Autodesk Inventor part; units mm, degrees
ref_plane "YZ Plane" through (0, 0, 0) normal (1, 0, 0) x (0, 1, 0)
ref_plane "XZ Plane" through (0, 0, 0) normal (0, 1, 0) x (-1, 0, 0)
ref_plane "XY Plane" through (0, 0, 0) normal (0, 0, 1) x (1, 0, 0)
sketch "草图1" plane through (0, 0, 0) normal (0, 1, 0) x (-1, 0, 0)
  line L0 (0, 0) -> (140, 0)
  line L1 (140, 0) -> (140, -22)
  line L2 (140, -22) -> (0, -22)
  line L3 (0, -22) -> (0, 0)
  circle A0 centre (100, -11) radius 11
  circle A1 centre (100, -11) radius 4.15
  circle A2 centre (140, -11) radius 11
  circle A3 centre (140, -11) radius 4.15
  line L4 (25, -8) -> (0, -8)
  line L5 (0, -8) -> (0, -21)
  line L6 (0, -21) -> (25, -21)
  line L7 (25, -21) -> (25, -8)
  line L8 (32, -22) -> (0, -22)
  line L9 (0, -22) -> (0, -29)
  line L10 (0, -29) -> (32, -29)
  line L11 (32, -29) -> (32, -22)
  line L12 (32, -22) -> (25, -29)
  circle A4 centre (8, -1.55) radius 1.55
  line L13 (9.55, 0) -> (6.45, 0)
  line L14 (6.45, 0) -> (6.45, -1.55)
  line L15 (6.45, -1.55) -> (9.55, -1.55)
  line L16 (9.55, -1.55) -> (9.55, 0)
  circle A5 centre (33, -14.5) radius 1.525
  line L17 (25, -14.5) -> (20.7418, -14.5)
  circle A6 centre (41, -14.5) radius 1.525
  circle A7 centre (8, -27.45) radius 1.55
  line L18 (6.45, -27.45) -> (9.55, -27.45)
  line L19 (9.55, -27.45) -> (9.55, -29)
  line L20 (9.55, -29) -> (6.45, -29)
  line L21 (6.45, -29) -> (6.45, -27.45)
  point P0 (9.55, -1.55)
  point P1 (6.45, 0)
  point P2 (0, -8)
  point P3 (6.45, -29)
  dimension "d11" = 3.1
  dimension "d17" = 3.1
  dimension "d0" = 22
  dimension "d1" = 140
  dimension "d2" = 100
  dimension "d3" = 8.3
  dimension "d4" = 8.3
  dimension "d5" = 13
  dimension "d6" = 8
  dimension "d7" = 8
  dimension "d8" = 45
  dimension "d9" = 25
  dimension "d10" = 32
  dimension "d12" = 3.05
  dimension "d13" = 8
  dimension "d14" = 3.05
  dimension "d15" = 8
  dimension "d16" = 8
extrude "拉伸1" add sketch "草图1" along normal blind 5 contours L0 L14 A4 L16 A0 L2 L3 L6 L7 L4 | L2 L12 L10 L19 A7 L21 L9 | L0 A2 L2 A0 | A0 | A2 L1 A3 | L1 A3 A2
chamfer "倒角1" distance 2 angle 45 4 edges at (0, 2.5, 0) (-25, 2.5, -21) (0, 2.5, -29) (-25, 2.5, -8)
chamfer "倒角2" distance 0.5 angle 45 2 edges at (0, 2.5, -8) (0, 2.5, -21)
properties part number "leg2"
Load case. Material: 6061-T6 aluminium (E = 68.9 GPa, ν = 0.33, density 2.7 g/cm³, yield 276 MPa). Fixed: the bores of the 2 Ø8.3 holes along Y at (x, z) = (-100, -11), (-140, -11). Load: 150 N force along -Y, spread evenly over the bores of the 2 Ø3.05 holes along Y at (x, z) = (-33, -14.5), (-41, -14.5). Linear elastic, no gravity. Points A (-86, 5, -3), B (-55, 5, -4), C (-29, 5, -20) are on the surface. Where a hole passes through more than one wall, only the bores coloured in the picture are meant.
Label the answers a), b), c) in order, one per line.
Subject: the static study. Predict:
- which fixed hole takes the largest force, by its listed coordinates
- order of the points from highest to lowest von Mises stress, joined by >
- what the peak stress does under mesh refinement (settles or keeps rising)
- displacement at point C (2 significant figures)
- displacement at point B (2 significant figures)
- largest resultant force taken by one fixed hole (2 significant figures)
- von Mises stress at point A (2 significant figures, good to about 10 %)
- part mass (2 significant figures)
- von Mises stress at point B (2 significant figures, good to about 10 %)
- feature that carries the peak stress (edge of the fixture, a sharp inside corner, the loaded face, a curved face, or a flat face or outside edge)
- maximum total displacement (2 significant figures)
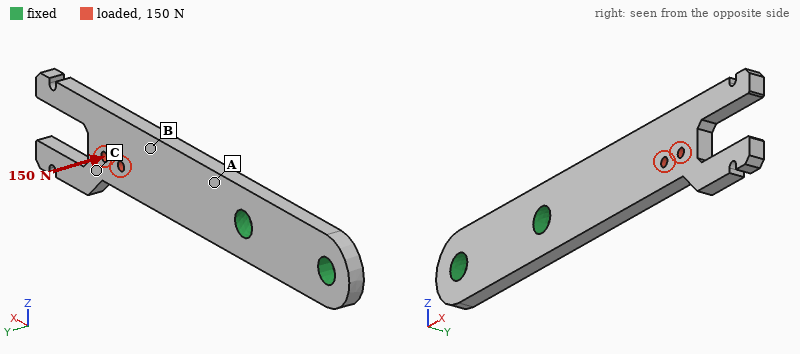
a) (-100, -11)
b) A > B > C
c) keeps rising
d) 0.84 mm
e) 0.39 mm
f) 150 N
g) 78 MPa
h) 41 g
i) 30 MPa
j) edge of the fixture
k) 1.4 mm
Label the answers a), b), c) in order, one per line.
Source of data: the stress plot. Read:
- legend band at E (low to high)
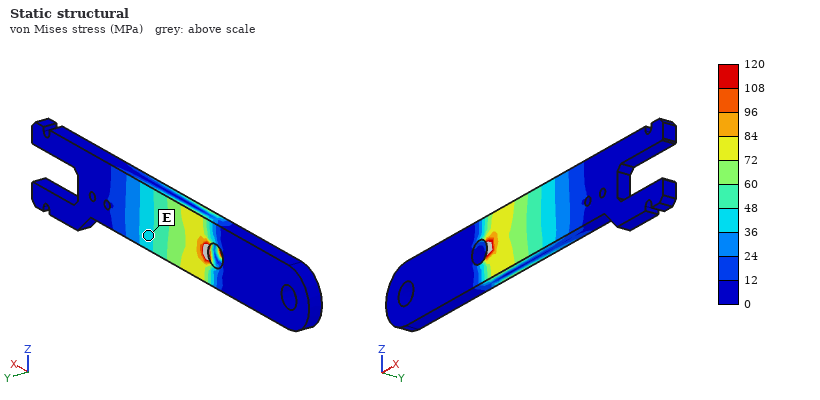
a) 36 to 48 MPa
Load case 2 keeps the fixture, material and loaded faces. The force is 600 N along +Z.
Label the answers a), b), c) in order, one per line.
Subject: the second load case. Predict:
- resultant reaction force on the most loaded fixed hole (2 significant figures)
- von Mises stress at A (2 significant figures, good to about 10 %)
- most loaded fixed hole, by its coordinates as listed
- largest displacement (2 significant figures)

a) 950 N
b) 51 MPa
c) (-100, -11)
d) 0.39 mm
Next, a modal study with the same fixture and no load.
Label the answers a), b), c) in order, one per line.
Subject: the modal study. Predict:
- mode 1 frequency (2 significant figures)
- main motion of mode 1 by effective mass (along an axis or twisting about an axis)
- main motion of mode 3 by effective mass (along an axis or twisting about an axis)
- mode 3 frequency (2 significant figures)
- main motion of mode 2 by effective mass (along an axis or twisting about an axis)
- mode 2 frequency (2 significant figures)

a) 490 Hz
b) along Y
c) twisting about X
d) 2300 Hz
e) along Z
f) 1700 Hz
